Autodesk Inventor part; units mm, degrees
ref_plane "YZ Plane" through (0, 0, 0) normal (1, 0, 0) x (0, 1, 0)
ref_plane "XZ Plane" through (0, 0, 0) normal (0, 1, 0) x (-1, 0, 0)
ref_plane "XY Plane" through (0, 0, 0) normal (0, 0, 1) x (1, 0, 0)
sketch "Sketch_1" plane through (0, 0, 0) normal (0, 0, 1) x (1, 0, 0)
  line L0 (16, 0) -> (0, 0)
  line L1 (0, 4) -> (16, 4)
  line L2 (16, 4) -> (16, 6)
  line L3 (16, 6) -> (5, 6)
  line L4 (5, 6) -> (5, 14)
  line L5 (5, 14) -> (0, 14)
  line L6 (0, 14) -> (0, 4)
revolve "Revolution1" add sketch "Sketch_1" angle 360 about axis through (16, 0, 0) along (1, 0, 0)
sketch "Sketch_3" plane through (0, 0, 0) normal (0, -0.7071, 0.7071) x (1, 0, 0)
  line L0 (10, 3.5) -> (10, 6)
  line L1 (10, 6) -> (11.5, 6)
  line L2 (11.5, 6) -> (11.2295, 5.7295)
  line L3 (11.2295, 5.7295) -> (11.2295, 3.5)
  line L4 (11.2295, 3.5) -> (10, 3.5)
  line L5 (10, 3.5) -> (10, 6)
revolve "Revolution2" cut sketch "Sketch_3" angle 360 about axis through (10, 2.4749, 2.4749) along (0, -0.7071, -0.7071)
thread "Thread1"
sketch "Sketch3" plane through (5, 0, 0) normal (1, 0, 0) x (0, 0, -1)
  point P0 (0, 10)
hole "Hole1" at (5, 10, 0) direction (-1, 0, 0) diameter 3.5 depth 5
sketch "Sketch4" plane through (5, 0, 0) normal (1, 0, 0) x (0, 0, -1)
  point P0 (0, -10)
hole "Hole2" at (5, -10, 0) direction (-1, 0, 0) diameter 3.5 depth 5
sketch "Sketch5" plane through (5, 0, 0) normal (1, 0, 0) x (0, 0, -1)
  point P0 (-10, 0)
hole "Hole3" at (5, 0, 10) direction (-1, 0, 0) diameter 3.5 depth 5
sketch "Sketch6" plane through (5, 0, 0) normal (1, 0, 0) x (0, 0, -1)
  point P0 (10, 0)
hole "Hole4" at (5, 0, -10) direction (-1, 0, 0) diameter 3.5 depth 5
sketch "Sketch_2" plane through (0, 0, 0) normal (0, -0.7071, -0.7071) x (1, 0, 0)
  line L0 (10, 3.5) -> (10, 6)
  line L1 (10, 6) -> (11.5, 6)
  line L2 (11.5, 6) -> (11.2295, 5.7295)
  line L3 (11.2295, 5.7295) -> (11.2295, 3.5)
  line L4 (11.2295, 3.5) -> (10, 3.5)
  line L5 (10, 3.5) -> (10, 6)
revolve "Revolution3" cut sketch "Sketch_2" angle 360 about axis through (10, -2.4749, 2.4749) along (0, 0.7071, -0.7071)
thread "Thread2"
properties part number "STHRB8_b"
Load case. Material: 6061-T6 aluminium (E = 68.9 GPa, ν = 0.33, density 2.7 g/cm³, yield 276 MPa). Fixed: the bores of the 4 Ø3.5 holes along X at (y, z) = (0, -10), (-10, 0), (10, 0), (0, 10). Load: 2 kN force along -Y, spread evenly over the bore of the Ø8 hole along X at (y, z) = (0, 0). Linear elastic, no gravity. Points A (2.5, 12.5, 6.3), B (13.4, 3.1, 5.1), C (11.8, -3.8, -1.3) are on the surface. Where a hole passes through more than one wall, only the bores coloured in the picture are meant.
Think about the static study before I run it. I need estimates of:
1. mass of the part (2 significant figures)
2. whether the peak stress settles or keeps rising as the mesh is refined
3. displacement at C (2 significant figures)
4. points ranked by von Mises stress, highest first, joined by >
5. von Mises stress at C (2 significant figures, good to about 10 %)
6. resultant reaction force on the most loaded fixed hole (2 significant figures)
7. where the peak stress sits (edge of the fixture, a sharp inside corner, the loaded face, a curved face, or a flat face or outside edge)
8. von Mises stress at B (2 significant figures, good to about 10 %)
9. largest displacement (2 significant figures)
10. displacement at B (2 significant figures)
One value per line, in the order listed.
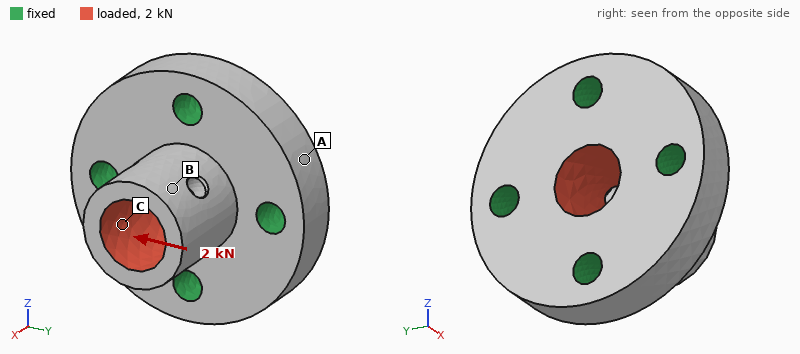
8.9 g
keeps rising
16 µm
C > B > A
25 MPa
870 N
a sharp inside corner
15 MPa
22 µm
18 µm
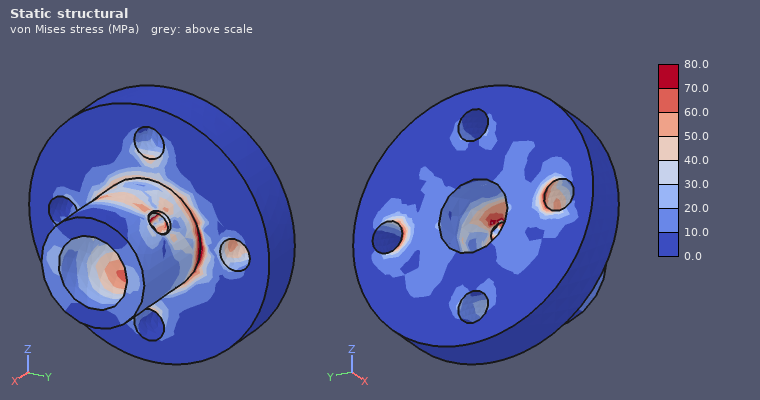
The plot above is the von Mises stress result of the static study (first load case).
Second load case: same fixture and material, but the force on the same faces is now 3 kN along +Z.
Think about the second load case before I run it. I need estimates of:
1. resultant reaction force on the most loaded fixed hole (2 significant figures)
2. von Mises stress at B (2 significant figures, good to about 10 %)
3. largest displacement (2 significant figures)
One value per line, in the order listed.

1.3 kN
30 MPa
34 µm
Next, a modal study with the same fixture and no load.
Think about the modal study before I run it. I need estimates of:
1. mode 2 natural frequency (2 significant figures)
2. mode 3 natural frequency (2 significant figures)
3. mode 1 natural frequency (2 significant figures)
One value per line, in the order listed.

34 kHz
54 kHz
34 kHz
